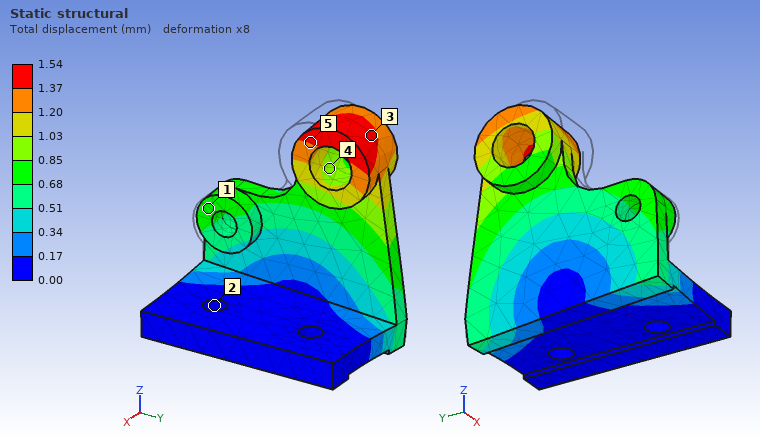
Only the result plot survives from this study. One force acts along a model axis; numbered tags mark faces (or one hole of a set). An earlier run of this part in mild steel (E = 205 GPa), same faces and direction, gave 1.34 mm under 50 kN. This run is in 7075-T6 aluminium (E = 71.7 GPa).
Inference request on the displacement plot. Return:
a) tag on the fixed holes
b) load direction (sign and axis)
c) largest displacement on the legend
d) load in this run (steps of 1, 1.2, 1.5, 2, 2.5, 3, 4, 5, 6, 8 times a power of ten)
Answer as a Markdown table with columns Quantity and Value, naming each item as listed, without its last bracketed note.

| Quantity | Value |
|---|---|
| tag on the fixed holes | 2 |
| load direction | +Y |
| largest displacement on the legend | 1.54 mm |
| load in this run | 20 kN |
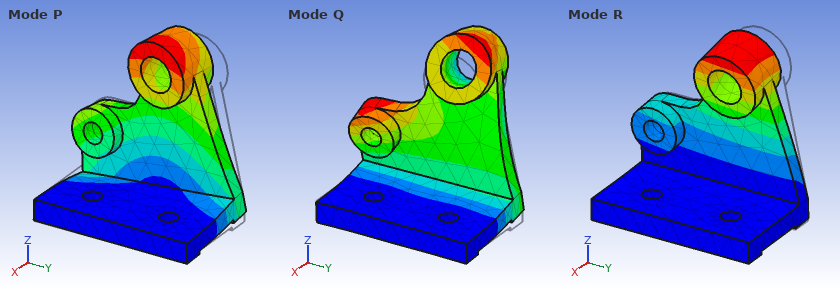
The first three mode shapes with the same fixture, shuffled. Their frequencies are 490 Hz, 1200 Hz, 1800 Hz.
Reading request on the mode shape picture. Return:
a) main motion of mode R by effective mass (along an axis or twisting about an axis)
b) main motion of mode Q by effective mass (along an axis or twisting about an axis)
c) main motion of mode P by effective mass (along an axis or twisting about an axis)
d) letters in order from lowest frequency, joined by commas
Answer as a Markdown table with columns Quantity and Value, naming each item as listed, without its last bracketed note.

| Quantity | Value |
|---|---|
| main motion of mode R by effective mass | along X |
| main motion of mode Q by effective mass | along Z |
| main motion of mode P by effective mass | along Y |
| letters in order from lowest frequency, joined by commas | R, P, Q |
